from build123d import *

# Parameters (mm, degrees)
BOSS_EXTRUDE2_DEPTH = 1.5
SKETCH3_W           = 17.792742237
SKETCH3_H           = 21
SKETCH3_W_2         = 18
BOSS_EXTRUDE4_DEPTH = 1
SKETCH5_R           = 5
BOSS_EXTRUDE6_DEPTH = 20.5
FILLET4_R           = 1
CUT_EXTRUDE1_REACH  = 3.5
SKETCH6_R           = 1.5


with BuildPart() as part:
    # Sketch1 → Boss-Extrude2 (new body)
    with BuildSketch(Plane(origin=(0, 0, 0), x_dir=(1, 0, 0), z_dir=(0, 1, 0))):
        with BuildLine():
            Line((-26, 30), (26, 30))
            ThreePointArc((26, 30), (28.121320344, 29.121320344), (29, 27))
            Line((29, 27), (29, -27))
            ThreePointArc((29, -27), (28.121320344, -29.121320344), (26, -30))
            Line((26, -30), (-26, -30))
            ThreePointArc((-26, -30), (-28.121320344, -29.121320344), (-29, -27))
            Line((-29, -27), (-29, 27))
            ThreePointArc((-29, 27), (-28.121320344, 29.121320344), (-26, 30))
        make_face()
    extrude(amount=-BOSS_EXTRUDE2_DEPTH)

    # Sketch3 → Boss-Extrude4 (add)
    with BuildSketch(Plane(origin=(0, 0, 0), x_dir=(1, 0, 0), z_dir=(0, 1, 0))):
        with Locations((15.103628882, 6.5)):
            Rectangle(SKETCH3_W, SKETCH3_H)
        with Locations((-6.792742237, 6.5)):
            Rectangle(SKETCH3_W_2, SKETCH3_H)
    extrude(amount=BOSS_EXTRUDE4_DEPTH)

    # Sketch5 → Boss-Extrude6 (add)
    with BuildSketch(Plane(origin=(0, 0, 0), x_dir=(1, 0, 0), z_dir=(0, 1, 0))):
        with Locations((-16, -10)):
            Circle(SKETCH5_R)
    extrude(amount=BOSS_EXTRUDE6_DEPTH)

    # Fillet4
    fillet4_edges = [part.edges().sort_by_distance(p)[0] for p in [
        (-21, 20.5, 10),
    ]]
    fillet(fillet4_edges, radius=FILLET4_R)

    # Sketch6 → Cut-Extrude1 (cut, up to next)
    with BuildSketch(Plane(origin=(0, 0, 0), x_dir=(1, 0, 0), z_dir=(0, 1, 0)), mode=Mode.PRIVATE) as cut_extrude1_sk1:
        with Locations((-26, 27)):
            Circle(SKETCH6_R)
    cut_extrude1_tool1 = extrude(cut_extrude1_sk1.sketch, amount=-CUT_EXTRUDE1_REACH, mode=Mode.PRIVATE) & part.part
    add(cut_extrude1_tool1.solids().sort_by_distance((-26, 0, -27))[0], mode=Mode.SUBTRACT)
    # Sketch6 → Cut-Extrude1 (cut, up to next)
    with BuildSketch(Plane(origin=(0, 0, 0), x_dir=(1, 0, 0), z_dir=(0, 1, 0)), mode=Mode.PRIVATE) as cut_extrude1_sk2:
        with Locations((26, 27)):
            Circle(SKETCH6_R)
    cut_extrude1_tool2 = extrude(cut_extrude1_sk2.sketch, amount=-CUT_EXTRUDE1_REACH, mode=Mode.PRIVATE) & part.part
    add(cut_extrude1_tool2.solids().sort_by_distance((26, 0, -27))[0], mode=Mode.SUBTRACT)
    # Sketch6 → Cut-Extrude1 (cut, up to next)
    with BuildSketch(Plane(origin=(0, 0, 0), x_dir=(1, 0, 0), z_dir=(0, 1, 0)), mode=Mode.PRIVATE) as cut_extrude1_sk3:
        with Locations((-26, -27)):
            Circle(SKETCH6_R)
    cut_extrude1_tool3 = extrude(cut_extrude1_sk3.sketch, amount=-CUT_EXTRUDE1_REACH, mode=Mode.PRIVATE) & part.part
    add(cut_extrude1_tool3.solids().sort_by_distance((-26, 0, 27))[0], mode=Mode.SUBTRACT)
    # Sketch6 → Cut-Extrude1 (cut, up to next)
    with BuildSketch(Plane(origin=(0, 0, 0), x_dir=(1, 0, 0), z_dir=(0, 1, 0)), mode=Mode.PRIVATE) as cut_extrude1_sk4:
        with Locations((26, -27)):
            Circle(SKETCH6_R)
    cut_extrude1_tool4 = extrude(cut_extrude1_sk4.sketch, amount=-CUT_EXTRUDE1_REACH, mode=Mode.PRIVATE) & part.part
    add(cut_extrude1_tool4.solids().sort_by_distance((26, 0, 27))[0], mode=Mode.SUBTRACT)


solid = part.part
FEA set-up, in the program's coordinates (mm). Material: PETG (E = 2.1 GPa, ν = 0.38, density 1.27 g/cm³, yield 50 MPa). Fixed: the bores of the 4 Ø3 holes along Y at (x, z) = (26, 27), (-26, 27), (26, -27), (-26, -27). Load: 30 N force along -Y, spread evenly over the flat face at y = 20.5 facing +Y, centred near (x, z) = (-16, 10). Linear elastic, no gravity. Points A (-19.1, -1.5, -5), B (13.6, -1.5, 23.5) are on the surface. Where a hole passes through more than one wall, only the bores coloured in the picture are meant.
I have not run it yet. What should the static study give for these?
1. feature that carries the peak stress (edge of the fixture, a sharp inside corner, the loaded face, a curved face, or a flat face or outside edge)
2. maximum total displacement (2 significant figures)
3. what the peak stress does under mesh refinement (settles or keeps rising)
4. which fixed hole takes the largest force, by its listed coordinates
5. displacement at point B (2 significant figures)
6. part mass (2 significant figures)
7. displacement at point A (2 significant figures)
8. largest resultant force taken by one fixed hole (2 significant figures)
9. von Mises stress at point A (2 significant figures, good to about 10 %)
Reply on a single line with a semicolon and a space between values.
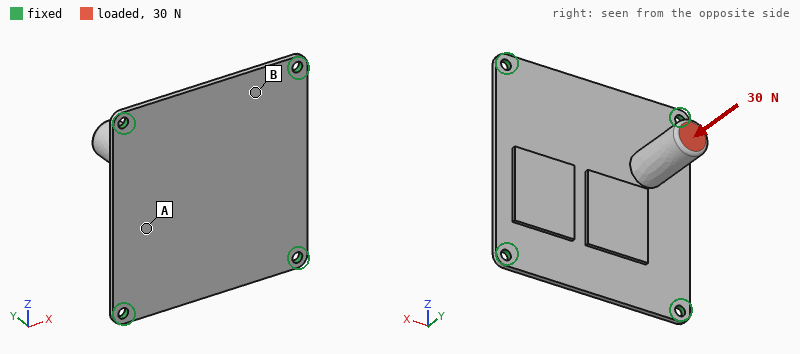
edge of the fixture; 1.0 mm; keeps rising; (-26, 27); 0.22 mm; 9.6 g; 0.76 mm; 19 N; 4.1 MPa
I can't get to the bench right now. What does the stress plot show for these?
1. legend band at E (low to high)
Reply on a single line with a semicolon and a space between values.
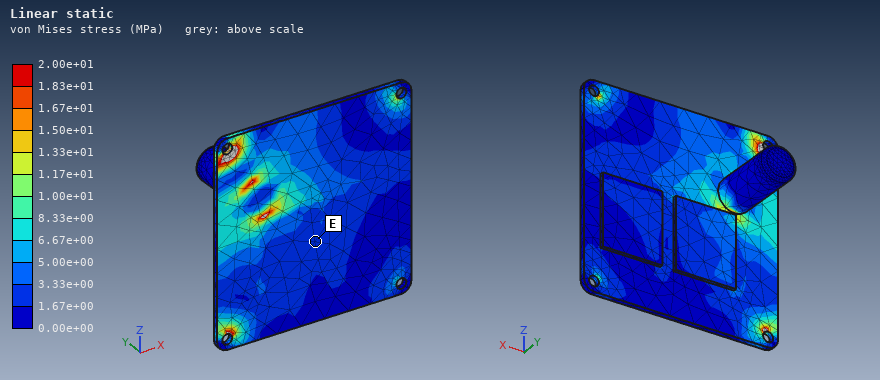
1.67e+00 to 3.33e+00 MPa
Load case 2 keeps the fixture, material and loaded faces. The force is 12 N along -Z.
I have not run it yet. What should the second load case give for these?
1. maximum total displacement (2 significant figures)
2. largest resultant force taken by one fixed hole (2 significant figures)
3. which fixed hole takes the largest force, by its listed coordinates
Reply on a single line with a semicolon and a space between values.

0.84 mm; 9.2 N; (-26, -27)
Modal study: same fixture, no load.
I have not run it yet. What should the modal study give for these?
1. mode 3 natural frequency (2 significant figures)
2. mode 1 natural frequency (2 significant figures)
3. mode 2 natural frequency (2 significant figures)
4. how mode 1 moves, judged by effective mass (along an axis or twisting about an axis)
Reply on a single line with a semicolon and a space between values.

790 Hz; 400 Hz; 540 Hz; along Y
